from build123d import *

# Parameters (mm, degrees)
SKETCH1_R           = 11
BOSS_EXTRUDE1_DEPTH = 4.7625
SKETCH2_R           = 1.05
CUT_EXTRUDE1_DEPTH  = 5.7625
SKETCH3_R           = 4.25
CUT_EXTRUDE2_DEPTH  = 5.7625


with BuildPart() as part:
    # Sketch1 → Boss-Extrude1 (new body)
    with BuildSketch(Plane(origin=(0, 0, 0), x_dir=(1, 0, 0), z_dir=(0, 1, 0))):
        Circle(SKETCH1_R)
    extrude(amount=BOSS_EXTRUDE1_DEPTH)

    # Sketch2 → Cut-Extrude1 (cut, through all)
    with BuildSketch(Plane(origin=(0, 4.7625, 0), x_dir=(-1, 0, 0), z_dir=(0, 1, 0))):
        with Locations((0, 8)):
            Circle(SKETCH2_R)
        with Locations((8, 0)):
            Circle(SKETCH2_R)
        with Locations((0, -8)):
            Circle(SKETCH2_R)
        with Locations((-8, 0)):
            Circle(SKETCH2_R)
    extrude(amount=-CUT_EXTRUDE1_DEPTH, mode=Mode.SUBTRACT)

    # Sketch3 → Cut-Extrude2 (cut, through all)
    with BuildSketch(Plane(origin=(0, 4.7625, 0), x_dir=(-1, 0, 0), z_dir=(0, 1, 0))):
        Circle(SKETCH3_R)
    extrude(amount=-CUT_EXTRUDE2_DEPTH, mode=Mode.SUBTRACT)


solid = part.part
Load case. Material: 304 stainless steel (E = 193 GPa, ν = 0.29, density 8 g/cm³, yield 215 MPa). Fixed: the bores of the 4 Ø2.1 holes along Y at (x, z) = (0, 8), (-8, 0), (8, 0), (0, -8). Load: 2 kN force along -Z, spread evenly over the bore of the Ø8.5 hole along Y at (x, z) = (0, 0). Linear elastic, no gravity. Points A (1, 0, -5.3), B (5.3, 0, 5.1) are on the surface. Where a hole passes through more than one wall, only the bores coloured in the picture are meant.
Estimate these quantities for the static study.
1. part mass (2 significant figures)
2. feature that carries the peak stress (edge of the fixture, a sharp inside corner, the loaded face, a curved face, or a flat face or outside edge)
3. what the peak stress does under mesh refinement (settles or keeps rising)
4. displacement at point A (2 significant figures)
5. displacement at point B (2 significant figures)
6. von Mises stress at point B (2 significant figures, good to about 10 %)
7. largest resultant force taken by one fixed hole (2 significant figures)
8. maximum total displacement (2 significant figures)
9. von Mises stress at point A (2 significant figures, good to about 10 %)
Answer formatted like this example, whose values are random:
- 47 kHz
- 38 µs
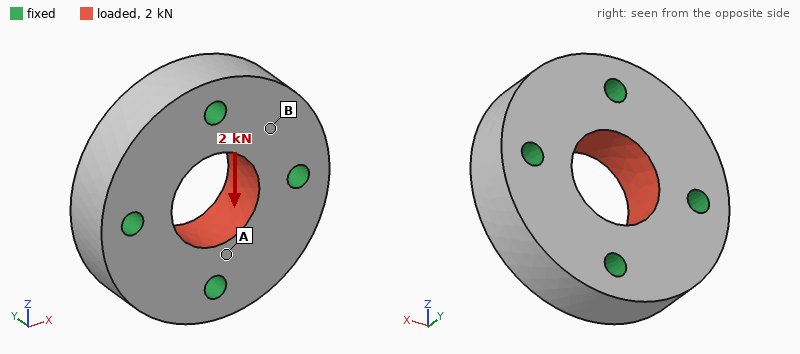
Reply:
- 12 g
- edge of the fixture
- keeps rising
- 0.28 µm
- 0.40 µm
- 7.6 MPa
- 550 N
- 0.63 µm
- 23 MPa
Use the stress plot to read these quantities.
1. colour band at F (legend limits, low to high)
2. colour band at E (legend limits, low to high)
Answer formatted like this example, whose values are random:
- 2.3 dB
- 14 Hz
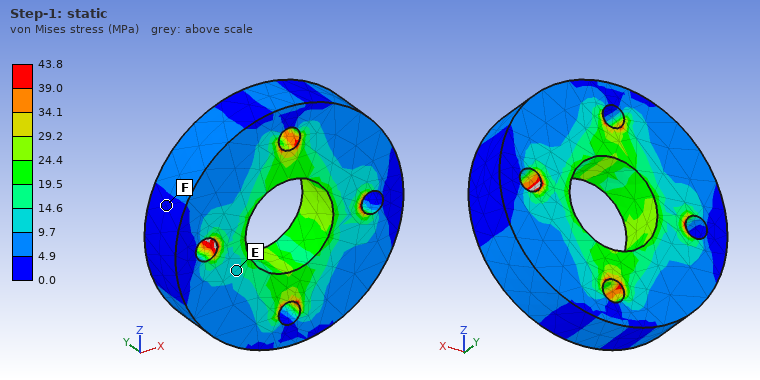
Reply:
- 0.0 to 4.9 MPa
- 9.7 to 14.6 MPa
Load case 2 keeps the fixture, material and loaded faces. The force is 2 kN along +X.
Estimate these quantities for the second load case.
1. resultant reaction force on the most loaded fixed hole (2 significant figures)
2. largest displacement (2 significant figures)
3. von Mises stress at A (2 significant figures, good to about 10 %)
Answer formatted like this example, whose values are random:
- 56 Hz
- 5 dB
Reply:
- 550 N
- 0.63 µm
- 14 MPa
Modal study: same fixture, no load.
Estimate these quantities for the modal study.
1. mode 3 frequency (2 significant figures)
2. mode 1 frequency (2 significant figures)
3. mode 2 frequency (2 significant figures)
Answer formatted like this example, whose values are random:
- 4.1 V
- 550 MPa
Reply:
- 83 kHz
- 79 kHz
- 83 kHz
